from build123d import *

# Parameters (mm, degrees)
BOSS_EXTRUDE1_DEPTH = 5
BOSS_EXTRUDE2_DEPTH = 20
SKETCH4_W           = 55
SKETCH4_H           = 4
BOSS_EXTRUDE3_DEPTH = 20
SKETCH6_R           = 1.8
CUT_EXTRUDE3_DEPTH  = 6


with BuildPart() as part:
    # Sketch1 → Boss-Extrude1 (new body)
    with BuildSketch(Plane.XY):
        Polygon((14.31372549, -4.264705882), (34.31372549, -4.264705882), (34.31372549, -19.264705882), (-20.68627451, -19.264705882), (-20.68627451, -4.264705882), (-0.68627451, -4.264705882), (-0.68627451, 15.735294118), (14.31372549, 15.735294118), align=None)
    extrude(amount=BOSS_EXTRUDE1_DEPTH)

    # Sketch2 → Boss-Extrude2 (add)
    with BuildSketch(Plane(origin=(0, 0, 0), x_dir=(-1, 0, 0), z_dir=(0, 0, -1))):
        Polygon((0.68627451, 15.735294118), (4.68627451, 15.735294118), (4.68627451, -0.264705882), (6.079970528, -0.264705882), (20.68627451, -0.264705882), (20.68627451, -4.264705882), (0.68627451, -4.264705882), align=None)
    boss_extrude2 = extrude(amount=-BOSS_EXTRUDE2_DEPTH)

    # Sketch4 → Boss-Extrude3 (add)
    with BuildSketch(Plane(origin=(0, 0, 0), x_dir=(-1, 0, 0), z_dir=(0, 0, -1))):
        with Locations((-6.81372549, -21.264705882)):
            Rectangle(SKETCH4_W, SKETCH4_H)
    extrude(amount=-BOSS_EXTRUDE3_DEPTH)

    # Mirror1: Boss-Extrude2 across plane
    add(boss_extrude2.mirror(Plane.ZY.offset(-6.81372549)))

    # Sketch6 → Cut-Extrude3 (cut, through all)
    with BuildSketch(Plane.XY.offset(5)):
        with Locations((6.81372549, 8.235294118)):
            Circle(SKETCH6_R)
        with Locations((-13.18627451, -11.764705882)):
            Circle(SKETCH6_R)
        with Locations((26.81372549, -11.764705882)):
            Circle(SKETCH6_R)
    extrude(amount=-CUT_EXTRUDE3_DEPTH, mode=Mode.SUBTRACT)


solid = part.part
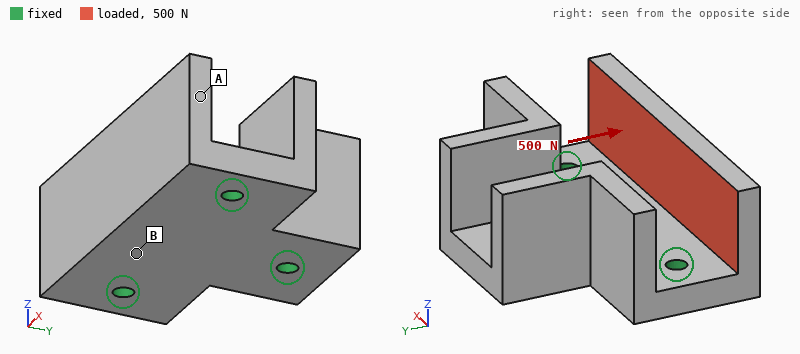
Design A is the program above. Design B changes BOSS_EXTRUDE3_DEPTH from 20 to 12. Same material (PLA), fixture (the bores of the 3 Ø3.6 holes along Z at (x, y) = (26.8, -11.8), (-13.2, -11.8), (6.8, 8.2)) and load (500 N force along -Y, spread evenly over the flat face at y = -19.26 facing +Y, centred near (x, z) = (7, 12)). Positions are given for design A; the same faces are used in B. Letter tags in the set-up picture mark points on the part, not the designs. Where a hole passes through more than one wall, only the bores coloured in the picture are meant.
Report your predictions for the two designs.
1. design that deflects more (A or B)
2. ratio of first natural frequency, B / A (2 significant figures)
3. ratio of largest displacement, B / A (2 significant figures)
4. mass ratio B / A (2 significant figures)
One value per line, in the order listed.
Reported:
A
1.4
0.33
0.89
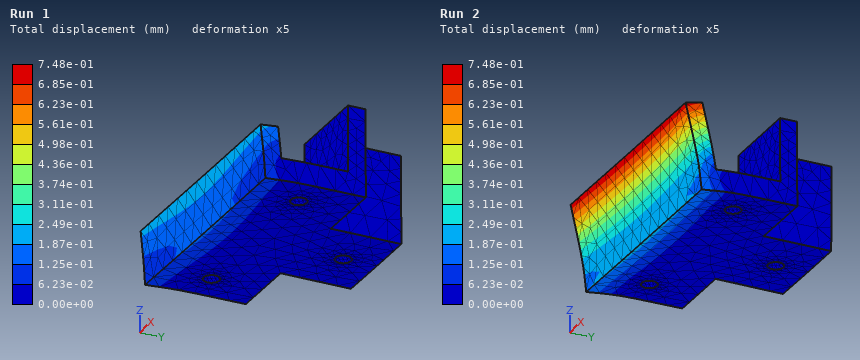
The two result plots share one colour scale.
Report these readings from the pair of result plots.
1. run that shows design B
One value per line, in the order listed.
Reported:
Run 1
